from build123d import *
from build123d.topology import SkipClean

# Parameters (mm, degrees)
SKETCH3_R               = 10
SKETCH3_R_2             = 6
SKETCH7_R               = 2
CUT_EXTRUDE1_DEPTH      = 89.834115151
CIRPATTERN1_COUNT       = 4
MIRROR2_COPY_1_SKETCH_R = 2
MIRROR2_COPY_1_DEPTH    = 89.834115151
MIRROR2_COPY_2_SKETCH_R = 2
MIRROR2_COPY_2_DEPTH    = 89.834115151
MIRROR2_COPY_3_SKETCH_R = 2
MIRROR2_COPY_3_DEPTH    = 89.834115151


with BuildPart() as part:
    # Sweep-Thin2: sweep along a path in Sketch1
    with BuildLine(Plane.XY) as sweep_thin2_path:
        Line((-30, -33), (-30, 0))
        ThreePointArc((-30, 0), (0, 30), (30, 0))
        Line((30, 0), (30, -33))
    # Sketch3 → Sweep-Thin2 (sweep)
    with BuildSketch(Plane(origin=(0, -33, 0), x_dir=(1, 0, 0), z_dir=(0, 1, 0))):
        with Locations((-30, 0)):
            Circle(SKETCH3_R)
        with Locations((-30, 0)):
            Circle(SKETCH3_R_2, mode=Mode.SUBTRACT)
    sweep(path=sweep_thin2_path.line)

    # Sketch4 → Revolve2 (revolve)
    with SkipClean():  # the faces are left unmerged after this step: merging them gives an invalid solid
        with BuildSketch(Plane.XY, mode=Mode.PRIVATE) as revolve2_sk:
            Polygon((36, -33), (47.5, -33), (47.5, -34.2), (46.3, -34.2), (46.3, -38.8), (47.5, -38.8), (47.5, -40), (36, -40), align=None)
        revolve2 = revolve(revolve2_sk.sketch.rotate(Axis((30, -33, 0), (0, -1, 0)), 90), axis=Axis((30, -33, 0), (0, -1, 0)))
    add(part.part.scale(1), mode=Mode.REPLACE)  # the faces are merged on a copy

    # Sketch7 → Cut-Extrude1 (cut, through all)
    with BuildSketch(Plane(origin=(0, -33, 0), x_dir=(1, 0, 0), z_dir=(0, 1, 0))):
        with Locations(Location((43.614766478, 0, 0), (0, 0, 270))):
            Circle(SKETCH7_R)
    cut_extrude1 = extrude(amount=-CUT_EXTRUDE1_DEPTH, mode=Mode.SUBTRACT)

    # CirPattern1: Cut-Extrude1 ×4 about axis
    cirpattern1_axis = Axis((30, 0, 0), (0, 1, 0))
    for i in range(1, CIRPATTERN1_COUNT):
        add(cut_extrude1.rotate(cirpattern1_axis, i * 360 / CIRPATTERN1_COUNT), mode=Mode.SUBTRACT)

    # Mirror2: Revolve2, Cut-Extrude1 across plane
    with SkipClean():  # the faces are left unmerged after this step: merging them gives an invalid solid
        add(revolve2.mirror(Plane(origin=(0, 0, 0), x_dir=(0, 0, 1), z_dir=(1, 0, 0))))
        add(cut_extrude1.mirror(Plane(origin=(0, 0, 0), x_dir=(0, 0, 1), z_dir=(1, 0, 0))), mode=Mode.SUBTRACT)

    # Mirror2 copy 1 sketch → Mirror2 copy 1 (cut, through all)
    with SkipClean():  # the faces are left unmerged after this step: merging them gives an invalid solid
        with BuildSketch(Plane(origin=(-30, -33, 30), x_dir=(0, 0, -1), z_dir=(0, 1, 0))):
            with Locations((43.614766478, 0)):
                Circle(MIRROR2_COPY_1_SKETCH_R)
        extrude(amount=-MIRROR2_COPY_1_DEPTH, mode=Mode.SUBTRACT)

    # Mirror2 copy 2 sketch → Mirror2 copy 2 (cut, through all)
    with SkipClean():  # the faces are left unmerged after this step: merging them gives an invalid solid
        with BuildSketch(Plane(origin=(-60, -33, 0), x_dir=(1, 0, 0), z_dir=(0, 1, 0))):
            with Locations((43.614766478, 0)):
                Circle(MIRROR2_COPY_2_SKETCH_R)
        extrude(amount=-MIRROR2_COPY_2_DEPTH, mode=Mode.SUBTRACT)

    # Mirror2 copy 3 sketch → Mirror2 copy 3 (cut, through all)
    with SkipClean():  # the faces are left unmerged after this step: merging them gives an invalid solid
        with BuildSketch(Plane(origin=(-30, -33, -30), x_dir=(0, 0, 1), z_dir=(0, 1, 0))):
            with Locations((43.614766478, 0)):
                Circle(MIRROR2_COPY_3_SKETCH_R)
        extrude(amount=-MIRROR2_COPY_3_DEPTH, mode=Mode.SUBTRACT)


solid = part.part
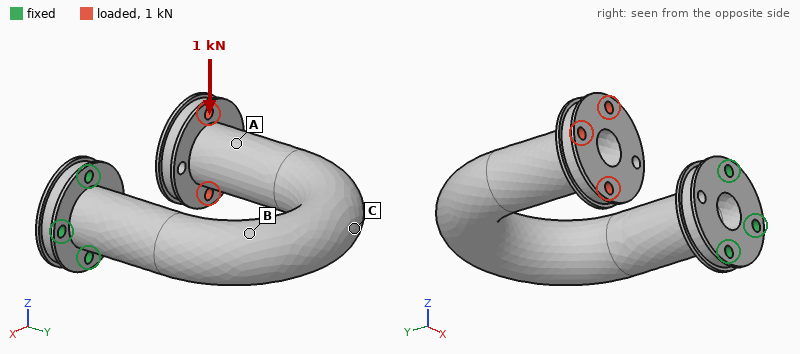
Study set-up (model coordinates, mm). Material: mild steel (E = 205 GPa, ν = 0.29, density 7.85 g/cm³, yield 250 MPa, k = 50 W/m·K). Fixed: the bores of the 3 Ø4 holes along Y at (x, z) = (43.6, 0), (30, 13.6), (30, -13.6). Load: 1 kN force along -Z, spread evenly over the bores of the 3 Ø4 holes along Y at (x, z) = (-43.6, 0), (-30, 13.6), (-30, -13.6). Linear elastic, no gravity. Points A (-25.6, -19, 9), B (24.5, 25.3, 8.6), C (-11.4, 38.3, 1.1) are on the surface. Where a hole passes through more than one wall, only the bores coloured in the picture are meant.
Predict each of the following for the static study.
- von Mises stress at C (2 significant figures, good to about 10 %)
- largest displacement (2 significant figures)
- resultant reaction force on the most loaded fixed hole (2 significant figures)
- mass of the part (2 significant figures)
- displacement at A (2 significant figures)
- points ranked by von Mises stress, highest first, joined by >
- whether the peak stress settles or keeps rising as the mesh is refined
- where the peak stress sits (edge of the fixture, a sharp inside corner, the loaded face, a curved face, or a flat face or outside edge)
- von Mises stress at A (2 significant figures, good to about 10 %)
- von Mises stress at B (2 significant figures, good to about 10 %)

53 MPa
0.65 mm
2.1 kN
330 g
0.43 mm
B > C > A
keeps rising
a sharp inside corner
21 MPa
86 MPa
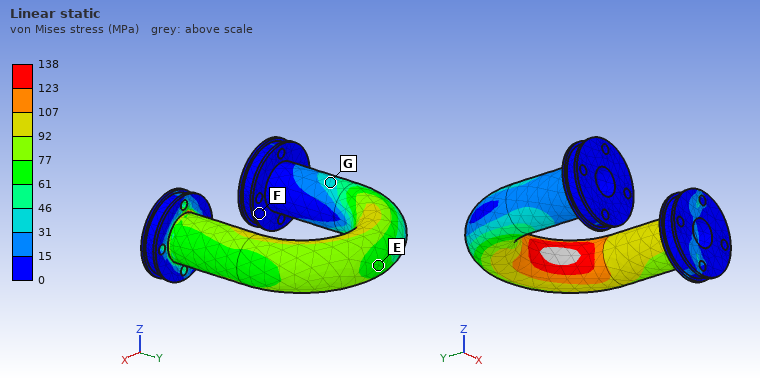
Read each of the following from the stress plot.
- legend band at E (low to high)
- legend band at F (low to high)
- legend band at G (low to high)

61 to 77 MPa
0 to 15 MPa
31 to 46 MPa
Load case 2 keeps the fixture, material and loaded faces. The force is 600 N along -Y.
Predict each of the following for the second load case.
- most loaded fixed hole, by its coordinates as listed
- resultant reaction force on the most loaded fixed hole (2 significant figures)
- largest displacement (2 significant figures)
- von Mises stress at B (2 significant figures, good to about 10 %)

(43.6, 0)
1.9 kN
0.25 mm
30 MPa
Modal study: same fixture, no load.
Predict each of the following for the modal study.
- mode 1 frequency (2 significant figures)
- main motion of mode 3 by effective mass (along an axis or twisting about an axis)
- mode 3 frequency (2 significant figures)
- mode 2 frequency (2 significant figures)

710 Hz
along X
1200 Hz
720 Hz
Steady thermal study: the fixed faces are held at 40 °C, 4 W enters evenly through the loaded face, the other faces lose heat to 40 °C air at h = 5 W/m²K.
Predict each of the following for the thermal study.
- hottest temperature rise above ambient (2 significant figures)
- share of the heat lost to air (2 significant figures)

43 K
51 %
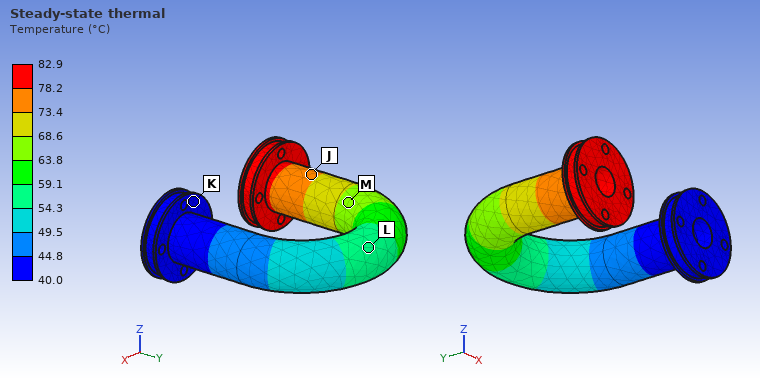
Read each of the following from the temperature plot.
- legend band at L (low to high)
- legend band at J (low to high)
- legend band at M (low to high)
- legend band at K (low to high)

54.3 to 59.1 °C
73.4 to 78.2 °C
63.8 to 68.6 °C
40.0 to 44.8 °C
